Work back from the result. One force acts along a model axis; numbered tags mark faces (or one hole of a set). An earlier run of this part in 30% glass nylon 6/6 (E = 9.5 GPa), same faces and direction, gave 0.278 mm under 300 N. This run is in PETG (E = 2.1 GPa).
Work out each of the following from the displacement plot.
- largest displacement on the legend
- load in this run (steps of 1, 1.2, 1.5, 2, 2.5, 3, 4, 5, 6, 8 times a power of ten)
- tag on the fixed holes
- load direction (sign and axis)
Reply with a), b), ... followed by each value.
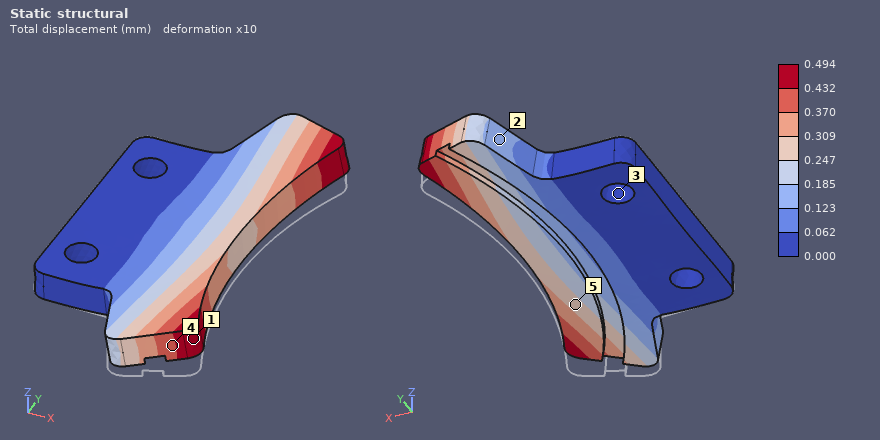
a) 0.494 mm
b) 120 N
c) 3
d) +Z
